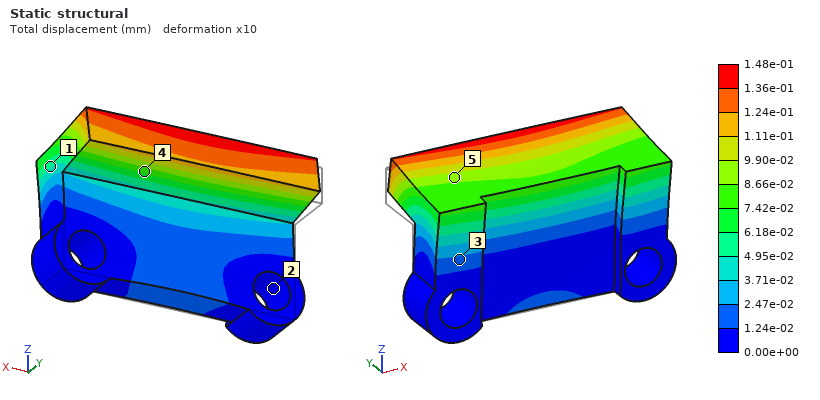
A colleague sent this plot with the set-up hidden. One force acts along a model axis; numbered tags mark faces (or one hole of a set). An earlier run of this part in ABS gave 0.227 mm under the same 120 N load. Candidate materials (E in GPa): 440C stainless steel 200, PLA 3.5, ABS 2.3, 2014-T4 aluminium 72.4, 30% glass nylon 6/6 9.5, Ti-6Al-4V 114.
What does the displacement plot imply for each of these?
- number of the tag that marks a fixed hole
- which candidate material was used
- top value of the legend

2
PLA
1.48e-01 mm
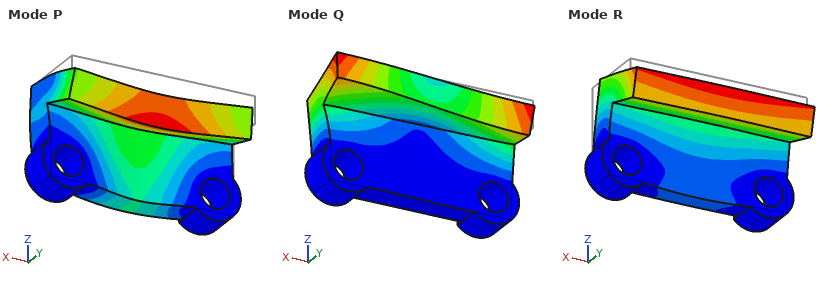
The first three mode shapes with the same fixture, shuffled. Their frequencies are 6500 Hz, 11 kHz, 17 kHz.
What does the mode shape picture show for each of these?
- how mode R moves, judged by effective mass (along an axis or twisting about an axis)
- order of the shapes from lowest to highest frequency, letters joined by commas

along Y
R, Q, P
